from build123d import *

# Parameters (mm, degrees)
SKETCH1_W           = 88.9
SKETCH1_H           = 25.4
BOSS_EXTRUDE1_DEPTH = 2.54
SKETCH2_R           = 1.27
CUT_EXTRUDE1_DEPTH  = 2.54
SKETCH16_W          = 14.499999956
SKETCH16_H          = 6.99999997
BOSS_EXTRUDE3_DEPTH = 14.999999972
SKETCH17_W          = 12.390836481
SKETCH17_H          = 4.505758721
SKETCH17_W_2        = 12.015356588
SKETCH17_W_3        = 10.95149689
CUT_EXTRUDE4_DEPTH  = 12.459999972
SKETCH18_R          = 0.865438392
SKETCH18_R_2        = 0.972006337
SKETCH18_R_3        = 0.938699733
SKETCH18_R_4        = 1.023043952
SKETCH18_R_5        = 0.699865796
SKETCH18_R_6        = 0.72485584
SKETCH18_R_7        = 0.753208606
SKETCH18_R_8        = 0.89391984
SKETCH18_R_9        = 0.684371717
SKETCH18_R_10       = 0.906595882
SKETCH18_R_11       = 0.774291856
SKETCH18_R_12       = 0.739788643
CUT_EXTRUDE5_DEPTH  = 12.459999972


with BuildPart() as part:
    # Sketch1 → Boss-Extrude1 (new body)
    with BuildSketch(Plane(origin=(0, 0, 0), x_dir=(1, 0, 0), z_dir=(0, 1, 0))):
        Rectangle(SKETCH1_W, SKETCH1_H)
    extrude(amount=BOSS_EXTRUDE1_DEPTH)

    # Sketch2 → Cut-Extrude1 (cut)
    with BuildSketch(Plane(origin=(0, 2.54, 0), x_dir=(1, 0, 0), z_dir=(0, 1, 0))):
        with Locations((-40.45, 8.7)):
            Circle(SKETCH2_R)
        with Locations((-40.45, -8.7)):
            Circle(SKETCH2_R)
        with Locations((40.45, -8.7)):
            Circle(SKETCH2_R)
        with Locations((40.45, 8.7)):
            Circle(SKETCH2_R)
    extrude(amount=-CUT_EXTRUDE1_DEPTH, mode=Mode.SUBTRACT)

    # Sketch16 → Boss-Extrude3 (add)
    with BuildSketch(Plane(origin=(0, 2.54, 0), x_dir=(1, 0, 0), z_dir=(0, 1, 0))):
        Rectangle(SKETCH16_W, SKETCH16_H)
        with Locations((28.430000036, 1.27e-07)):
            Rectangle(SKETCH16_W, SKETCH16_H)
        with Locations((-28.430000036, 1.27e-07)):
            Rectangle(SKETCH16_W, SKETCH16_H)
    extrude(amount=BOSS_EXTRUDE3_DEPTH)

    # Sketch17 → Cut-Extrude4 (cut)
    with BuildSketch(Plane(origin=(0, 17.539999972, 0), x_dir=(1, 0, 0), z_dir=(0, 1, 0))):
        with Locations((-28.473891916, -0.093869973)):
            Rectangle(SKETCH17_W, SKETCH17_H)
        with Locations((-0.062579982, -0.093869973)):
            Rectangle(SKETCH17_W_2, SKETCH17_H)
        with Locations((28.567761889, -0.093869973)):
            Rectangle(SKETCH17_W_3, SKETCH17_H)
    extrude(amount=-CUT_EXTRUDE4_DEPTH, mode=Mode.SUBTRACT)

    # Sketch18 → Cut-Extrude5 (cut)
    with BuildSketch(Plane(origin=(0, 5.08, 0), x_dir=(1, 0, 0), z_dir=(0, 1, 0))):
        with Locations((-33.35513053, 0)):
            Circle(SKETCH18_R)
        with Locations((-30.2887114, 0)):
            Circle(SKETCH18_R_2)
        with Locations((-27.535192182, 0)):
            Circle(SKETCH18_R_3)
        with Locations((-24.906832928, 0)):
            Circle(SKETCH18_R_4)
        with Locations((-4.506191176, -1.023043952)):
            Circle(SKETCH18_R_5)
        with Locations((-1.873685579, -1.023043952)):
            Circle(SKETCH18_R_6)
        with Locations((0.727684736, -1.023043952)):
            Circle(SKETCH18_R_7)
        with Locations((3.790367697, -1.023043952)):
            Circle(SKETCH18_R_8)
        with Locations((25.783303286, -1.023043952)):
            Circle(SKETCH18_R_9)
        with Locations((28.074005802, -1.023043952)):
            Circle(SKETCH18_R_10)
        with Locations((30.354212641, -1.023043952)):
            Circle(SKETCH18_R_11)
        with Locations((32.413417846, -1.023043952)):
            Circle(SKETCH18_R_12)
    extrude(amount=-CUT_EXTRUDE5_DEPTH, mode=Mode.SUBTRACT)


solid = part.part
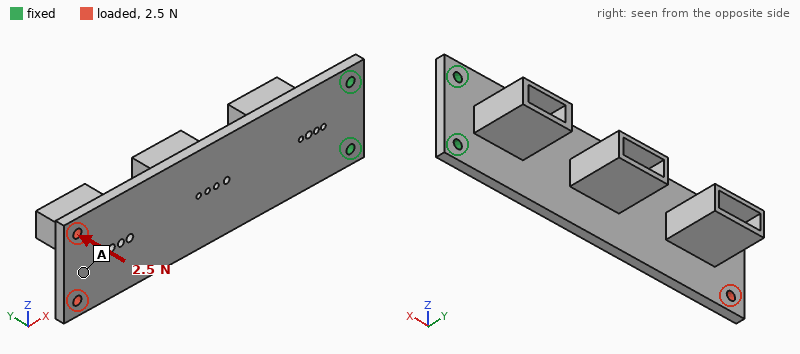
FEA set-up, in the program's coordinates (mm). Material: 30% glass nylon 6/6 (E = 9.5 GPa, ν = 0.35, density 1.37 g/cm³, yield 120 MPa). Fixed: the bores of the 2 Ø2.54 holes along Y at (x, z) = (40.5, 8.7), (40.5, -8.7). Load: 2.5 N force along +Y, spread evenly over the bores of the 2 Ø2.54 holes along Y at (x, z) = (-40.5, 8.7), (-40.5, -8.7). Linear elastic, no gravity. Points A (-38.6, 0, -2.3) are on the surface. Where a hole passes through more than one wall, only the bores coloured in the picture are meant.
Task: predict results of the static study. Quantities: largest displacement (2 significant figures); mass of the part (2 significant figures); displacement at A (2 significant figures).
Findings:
1.0 mm
11 g
0.91 mm
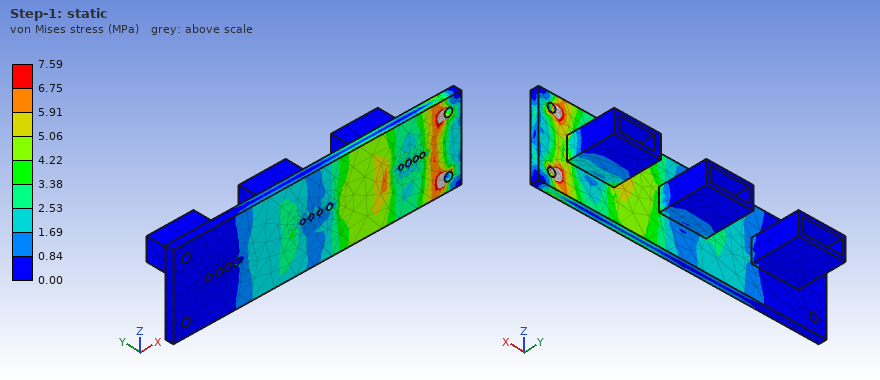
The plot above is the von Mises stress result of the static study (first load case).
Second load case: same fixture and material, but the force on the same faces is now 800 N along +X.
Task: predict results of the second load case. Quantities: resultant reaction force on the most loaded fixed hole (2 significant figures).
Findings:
410 N
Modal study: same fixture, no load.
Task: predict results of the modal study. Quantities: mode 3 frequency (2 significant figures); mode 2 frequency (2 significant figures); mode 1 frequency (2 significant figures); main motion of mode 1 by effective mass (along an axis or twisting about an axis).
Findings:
900 Hz
890 Hz
150 Hz
along Y
